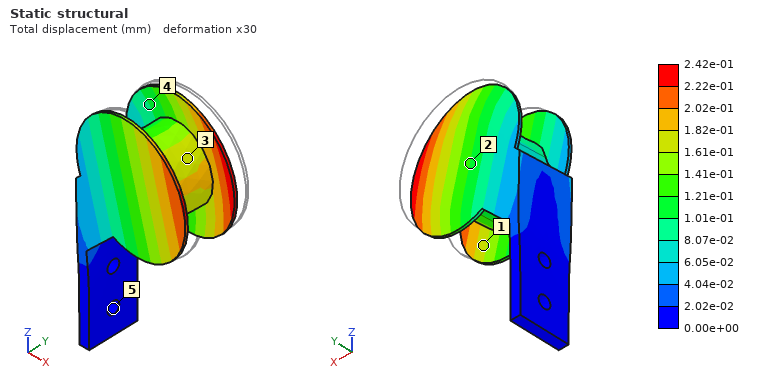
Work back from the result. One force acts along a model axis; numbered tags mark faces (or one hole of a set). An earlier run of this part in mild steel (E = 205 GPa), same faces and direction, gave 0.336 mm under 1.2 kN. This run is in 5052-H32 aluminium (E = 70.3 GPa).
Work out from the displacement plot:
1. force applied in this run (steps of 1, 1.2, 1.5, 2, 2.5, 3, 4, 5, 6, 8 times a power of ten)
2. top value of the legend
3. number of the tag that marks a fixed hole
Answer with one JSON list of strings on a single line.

["300 N", "2.42e-01 mm", "5"]
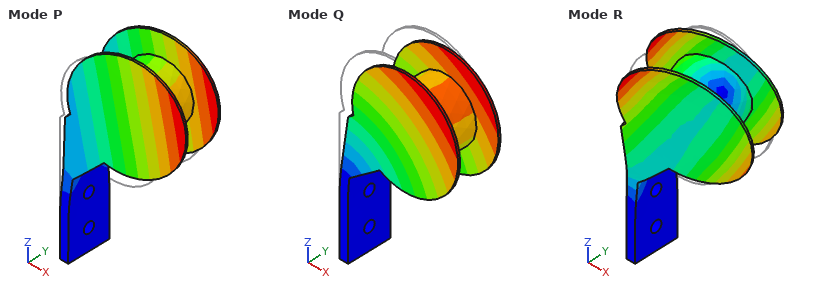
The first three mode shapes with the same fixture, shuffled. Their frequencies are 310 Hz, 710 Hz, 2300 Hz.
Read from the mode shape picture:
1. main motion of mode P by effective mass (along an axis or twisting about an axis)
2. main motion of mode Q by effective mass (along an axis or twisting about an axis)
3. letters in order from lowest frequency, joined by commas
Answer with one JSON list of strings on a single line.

["along Y", "along X", "Q, P, R"]
